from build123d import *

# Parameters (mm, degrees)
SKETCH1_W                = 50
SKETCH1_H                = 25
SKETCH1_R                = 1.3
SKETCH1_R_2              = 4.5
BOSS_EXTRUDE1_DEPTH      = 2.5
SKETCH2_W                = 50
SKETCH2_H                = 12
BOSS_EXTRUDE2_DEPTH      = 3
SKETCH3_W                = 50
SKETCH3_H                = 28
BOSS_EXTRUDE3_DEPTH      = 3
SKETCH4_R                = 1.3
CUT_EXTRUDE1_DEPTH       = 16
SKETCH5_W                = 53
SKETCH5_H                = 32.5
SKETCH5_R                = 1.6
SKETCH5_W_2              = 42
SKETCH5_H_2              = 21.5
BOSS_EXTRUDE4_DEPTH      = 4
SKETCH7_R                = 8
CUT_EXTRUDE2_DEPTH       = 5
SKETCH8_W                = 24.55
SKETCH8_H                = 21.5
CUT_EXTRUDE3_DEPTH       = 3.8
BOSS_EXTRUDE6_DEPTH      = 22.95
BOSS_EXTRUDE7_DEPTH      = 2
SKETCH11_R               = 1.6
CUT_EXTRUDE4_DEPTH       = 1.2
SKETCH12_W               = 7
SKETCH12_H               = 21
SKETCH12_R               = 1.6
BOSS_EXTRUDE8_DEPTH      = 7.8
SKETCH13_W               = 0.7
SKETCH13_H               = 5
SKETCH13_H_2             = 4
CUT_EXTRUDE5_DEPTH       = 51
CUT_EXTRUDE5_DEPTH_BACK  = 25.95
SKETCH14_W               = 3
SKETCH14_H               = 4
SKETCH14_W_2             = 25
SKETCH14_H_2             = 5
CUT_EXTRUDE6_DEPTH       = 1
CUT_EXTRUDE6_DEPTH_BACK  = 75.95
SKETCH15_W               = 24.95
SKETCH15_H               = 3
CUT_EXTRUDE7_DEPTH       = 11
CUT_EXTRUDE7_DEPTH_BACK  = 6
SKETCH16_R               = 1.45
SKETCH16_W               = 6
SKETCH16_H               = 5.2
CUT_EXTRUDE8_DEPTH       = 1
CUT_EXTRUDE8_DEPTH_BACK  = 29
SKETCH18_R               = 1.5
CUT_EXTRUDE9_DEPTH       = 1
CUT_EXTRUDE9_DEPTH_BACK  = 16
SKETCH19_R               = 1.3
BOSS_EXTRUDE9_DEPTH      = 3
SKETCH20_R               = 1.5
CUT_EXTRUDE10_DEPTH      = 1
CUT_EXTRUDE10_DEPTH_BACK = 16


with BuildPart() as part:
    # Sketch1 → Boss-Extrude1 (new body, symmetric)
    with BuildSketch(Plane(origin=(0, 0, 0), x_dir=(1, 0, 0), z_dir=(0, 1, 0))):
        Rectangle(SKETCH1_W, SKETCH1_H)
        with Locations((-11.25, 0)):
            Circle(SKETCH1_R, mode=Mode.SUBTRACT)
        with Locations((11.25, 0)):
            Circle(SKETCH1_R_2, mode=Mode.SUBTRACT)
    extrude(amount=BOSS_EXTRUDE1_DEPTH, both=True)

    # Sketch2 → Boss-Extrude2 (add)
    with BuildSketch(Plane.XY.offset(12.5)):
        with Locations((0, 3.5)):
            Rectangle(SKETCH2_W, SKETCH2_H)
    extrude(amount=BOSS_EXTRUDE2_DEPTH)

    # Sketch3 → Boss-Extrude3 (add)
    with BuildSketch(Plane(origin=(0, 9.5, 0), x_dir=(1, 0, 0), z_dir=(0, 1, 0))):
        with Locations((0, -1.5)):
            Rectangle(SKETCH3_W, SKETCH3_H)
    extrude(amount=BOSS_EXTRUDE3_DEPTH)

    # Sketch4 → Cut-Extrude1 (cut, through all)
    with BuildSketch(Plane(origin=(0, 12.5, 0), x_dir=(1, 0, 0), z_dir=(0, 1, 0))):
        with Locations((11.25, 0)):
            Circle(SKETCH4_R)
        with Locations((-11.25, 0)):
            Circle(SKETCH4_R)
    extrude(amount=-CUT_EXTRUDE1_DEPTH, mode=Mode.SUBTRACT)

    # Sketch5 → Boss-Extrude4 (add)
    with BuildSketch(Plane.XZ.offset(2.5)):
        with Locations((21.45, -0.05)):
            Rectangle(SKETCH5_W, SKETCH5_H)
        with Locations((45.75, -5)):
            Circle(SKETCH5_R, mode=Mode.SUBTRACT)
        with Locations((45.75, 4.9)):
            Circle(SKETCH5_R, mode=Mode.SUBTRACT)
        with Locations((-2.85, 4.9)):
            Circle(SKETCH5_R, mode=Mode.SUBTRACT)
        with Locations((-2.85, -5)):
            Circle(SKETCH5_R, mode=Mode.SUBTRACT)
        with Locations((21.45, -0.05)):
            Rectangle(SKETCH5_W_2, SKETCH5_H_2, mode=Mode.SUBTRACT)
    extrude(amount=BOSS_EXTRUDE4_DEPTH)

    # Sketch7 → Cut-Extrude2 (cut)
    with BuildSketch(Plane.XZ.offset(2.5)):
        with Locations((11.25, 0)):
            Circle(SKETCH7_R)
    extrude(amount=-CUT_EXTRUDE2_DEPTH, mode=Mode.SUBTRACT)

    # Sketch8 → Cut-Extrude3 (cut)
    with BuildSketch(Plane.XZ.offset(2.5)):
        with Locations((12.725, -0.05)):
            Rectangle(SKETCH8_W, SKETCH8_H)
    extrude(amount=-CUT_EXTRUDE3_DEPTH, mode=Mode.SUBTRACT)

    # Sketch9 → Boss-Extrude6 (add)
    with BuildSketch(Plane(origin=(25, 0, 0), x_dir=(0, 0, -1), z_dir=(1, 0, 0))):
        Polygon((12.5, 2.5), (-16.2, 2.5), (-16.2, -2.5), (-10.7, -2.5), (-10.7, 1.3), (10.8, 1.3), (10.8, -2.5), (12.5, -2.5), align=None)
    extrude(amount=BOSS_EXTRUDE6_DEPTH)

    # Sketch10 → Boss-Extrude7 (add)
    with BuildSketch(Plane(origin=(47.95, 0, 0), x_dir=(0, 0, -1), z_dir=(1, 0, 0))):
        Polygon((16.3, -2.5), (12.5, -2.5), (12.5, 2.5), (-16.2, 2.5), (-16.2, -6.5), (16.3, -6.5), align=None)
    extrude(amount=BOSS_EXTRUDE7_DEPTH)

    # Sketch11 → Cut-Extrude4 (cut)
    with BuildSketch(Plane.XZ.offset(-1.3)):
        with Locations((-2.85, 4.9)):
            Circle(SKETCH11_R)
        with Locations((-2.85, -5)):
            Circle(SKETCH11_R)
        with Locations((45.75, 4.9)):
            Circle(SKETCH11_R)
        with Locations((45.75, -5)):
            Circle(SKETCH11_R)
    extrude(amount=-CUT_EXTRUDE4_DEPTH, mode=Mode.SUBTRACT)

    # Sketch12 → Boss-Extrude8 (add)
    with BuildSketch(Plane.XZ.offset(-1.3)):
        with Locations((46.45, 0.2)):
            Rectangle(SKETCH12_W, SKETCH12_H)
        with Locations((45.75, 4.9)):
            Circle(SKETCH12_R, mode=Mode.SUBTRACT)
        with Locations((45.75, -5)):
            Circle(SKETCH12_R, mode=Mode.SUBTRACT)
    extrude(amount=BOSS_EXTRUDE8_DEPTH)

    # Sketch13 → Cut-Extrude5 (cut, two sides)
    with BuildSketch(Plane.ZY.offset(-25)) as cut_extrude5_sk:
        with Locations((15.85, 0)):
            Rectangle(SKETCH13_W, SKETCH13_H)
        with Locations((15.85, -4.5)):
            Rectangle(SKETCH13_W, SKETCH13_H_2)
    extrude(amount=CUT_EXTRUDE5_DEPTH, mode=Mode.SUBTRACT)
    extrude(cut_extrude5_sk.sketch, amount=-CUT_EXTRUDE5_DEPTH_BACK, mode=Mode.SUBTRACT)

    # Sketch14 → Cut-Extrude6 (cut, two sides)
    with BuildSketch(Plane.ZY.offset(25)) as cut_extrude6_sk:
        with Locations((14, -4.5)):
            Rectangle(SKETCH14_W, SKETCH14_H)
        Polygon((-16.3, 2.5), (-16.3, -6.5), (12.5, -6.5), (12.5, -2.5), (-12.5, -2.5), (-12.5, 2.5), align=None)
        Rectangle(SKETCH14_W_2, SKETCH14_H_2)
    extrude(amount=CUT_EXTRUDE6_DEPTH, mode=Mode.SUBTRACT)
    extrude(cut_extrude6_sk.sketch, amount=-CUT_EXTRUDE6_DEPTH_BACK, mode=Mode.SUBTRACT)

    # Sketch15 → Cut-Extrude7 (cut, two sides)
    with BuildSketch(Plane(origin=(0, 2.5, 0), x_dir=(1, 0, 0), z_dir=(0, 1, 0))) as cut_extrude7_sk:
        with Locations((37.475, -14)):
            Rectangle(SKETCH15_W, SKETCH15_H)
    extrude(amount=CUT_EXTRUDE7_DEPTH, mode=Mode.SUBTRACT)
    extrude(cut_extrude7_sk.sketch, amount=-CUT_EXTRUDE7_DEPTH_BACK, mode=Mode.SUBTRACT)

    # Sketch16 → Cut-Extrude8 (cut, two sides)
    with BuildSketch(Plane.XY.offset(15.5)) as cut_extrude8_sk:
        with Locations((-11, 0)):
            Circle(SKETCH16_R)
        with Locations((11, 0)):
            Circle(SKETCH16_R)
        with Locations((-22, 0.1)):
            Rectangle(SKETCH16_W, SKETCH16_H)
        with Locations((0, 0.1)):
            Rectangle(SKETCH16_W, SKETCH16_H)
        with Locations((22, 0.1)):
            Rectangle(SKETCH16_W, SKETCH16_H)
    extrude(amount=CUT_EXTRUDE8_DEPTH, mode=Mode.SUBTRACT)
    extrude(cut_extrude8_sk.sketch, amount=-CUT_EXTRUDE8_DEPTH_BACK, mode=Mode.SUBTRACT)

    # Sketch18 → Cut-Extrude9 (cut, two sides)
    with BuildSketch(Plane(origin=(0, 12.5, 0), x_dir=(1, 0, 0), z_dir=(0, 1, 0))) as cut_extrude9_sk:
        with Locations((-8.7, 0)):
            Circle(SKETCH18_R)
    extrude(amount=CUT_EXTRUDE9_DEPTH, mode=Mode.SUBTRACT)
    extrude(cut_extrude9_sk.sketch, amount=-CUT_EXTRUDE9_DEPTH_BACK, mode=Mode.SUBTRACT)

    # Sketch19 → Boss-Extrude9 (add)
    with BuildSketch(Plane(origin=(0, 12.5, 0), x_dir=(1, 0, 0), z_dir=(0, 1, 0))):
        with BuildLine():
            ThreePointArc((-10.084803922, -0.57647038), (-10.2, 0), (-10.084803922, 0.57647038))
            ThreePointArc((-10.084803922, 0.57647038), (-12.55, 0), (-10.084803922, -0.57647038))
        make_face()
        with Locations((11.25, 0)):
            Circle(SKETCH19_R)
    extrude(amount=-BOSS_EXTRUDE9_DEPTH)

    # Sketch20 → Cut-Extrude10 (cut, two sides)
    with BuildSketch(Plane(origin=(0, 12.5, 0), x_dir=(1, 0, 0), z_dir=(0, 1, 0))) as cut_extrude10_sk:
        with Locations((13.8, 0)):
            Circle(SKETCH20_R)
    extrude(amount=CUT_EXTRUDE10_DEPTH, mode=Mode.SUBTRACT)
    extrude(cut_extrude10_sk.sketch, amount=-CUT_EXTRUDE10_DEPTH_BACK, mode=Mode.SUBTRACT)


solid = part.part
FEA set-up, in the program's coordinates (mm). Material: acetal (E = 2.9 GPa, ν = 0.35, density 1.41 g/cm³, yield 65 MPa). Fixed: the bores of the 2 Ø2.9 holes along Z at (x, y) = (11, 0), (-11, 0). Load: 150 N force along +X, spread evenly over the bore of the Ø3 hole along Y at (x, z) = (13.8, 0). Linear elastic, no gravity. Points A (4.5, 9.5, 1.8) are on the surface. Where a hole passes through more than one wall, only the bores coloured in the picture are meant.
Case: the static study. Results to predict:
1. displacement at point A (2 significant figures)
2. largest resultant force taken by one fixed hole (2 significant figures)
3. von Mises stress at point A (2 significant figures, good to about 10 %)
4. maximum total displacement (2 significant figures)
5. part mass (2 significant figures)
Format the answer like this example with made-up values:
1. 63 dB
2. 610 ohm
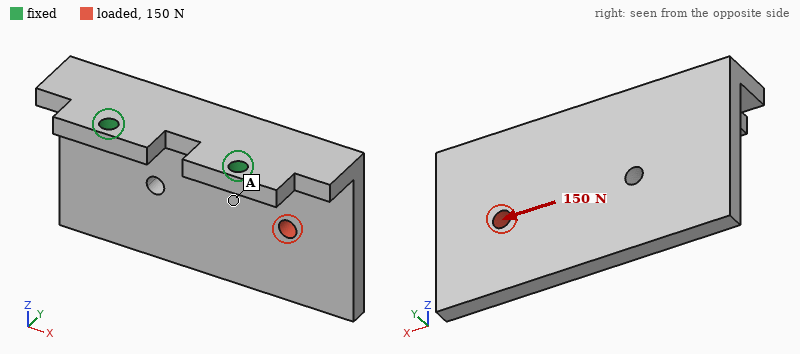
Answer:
1. 0.26 mm
2. 130 N
3. 5.2 MPa
4. 0.70 mm
5. 7.9 g
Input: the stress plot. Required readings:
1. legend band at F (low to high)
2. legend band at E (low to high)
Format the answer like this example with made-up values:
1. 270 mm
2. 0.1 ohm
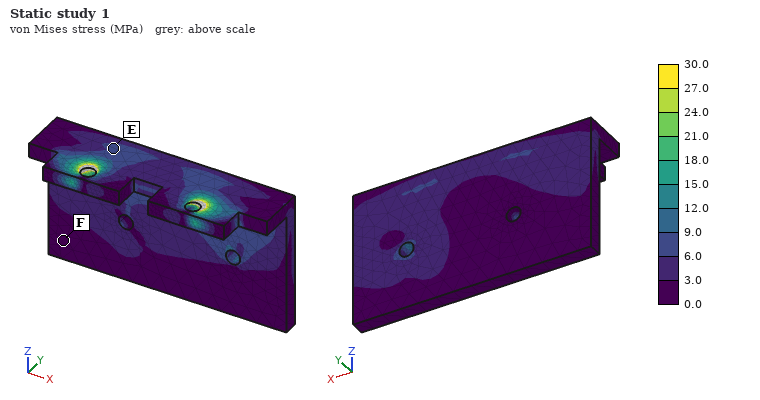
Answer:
1. 0.0 to 3.0 MPa
2. 6.0 to 9.0 MPa
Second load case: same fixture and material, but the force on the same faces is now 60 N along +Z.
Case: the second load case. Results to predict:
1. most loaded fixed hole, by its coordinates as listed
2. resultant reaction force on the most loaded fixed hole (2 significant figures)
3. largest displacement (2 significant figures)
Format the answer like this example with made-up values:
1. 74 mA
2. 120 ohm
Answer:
1. (11, 0)
2. 61 N
3. 0.71 mm
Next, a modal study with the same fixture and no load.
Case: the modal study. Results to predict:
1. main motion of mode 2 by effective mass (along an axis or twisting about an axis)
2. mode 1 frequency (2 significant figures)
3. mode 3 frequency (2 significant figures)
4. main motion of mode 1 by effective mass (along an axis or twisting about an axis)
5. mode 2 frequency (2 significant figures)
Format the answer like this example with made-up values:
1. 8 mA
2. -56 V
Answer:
1. along X
2. 540 Hz
3. 1500 Hz
4. along Y
5. 960 Hz
